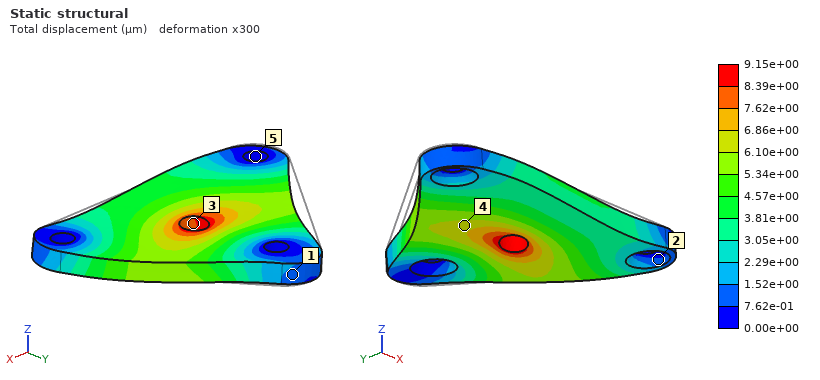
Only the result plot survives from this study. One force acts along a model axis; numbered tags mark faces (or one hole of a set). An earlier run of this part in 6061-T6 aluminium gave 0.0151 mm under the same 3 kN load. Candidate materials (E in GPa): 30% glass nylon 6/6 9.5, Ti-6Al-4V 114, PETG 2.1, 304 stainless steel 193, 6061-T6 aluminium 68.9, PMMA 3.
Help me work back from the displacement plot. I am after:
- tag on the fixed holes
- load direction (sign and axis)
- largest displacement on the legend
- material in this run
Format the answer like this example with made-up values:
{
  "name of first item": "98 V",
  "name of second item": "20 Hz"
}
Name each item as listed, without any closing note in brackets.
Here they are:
{
  "tag on the fixed holes": "5",
  "load direction": "+X",
  "largest displacement on the legend": "9.15e+00 µm",
  "material in this run": "Ti-6Al-4V"
}
